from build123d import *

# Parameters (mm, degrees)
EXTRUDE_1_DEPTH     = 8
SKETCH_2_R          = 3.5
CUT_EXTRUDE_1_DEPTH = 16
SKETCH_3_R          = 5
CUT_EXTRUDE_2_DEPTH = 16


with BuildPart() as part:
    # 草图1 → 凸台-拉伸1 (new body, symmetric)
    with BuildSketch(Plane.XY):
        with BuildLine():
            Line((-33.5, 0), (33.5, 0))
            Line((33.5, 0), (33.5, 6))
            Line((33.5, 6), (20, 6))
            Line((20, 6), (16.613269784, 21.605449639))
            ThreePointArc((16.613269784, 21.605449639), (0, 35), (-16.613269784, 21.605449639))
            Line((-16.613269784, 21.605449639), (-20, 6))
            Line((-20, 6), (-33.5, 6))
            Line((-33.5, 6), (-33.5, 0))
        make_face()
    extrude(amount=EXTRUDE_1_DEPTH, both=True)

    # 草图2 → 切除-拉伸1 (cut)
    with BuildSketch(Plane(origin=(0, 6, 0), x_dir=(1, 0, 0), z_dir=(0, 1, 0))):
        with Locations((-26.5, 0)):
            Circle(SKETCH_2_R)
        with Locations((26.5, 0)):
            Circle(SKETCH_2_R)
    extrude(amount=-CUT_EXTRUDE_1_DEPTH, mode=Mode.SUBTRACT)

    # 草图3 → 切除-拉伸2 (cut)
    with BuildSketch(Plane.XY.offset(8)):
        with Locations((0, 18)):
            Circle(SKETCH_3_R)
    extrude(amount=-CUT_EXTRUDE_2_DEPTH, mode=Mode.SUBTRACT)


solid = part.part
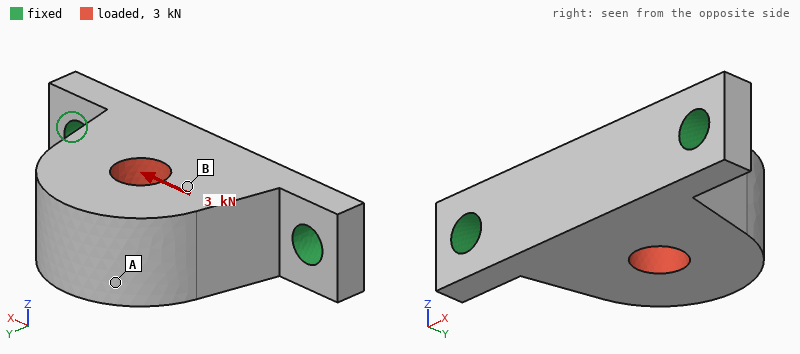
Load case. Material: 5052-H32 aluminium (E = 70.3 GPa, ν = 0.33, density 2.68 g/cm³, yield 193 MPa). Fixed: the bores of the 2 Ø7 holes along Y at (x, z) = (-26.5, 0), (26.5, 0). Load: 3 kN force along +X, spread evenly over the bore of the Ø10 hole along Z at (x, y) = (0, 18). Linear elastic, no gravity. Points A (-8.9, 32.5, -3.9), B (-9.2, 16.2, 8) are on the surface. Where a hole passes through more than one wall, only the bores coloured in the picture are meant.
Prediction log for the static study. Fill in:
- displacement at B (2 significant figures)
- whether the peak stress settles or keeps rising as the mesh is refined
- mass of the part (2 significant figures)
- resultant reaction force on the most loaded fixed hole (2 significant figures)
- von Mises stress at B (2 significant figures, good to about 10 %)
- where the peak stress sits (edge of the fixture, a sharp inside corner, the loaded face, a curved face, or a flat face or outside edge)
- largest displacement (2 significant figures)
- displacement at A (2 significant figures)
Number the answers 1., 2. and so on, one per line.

1. 7.1 µm
2. keeps rising
3. 51 g
4. 1.8 kN
5. 12 MPa
6. edge of the fixture
7. 12 µm
8. 12 µm
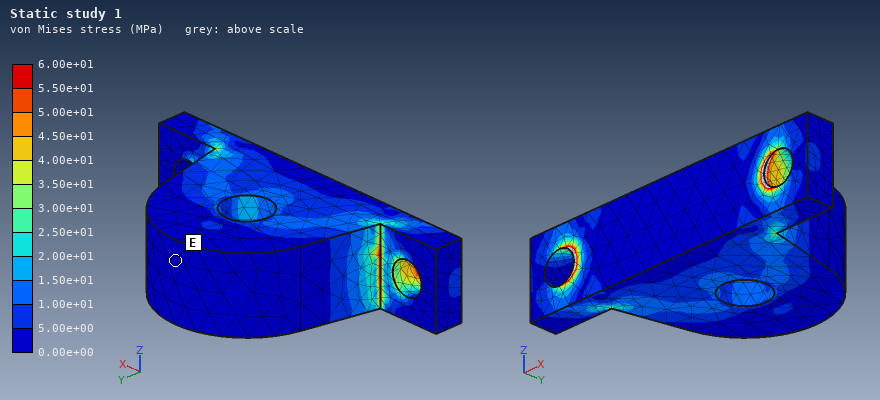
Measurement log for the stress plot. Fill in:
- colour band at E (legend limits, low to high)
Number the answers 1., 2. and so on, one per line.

1. 0.00e+00 to 5.00e+00 MPa
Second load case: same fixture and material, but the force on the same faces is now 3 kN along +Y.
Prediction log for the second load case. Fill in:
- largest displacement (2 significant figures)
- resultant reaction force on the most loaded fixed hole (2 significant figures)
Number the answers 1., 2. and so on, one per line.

1. 12 µm
2. 1.7 kN
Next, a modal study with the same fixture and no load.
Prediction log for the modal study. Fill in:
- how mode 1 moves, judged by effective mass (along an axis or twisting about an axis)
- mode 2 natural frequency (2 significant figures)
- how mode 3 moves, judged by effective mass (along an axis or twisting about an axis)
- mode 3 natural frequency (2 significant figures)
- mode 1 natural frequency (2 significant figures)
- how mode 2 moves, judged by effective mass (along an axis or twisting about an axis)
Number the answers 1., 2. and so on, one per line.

1. along Z
2. 13 kHz
3. along X
4. 14 kHz
5. 4100 Hz
6. along Y
